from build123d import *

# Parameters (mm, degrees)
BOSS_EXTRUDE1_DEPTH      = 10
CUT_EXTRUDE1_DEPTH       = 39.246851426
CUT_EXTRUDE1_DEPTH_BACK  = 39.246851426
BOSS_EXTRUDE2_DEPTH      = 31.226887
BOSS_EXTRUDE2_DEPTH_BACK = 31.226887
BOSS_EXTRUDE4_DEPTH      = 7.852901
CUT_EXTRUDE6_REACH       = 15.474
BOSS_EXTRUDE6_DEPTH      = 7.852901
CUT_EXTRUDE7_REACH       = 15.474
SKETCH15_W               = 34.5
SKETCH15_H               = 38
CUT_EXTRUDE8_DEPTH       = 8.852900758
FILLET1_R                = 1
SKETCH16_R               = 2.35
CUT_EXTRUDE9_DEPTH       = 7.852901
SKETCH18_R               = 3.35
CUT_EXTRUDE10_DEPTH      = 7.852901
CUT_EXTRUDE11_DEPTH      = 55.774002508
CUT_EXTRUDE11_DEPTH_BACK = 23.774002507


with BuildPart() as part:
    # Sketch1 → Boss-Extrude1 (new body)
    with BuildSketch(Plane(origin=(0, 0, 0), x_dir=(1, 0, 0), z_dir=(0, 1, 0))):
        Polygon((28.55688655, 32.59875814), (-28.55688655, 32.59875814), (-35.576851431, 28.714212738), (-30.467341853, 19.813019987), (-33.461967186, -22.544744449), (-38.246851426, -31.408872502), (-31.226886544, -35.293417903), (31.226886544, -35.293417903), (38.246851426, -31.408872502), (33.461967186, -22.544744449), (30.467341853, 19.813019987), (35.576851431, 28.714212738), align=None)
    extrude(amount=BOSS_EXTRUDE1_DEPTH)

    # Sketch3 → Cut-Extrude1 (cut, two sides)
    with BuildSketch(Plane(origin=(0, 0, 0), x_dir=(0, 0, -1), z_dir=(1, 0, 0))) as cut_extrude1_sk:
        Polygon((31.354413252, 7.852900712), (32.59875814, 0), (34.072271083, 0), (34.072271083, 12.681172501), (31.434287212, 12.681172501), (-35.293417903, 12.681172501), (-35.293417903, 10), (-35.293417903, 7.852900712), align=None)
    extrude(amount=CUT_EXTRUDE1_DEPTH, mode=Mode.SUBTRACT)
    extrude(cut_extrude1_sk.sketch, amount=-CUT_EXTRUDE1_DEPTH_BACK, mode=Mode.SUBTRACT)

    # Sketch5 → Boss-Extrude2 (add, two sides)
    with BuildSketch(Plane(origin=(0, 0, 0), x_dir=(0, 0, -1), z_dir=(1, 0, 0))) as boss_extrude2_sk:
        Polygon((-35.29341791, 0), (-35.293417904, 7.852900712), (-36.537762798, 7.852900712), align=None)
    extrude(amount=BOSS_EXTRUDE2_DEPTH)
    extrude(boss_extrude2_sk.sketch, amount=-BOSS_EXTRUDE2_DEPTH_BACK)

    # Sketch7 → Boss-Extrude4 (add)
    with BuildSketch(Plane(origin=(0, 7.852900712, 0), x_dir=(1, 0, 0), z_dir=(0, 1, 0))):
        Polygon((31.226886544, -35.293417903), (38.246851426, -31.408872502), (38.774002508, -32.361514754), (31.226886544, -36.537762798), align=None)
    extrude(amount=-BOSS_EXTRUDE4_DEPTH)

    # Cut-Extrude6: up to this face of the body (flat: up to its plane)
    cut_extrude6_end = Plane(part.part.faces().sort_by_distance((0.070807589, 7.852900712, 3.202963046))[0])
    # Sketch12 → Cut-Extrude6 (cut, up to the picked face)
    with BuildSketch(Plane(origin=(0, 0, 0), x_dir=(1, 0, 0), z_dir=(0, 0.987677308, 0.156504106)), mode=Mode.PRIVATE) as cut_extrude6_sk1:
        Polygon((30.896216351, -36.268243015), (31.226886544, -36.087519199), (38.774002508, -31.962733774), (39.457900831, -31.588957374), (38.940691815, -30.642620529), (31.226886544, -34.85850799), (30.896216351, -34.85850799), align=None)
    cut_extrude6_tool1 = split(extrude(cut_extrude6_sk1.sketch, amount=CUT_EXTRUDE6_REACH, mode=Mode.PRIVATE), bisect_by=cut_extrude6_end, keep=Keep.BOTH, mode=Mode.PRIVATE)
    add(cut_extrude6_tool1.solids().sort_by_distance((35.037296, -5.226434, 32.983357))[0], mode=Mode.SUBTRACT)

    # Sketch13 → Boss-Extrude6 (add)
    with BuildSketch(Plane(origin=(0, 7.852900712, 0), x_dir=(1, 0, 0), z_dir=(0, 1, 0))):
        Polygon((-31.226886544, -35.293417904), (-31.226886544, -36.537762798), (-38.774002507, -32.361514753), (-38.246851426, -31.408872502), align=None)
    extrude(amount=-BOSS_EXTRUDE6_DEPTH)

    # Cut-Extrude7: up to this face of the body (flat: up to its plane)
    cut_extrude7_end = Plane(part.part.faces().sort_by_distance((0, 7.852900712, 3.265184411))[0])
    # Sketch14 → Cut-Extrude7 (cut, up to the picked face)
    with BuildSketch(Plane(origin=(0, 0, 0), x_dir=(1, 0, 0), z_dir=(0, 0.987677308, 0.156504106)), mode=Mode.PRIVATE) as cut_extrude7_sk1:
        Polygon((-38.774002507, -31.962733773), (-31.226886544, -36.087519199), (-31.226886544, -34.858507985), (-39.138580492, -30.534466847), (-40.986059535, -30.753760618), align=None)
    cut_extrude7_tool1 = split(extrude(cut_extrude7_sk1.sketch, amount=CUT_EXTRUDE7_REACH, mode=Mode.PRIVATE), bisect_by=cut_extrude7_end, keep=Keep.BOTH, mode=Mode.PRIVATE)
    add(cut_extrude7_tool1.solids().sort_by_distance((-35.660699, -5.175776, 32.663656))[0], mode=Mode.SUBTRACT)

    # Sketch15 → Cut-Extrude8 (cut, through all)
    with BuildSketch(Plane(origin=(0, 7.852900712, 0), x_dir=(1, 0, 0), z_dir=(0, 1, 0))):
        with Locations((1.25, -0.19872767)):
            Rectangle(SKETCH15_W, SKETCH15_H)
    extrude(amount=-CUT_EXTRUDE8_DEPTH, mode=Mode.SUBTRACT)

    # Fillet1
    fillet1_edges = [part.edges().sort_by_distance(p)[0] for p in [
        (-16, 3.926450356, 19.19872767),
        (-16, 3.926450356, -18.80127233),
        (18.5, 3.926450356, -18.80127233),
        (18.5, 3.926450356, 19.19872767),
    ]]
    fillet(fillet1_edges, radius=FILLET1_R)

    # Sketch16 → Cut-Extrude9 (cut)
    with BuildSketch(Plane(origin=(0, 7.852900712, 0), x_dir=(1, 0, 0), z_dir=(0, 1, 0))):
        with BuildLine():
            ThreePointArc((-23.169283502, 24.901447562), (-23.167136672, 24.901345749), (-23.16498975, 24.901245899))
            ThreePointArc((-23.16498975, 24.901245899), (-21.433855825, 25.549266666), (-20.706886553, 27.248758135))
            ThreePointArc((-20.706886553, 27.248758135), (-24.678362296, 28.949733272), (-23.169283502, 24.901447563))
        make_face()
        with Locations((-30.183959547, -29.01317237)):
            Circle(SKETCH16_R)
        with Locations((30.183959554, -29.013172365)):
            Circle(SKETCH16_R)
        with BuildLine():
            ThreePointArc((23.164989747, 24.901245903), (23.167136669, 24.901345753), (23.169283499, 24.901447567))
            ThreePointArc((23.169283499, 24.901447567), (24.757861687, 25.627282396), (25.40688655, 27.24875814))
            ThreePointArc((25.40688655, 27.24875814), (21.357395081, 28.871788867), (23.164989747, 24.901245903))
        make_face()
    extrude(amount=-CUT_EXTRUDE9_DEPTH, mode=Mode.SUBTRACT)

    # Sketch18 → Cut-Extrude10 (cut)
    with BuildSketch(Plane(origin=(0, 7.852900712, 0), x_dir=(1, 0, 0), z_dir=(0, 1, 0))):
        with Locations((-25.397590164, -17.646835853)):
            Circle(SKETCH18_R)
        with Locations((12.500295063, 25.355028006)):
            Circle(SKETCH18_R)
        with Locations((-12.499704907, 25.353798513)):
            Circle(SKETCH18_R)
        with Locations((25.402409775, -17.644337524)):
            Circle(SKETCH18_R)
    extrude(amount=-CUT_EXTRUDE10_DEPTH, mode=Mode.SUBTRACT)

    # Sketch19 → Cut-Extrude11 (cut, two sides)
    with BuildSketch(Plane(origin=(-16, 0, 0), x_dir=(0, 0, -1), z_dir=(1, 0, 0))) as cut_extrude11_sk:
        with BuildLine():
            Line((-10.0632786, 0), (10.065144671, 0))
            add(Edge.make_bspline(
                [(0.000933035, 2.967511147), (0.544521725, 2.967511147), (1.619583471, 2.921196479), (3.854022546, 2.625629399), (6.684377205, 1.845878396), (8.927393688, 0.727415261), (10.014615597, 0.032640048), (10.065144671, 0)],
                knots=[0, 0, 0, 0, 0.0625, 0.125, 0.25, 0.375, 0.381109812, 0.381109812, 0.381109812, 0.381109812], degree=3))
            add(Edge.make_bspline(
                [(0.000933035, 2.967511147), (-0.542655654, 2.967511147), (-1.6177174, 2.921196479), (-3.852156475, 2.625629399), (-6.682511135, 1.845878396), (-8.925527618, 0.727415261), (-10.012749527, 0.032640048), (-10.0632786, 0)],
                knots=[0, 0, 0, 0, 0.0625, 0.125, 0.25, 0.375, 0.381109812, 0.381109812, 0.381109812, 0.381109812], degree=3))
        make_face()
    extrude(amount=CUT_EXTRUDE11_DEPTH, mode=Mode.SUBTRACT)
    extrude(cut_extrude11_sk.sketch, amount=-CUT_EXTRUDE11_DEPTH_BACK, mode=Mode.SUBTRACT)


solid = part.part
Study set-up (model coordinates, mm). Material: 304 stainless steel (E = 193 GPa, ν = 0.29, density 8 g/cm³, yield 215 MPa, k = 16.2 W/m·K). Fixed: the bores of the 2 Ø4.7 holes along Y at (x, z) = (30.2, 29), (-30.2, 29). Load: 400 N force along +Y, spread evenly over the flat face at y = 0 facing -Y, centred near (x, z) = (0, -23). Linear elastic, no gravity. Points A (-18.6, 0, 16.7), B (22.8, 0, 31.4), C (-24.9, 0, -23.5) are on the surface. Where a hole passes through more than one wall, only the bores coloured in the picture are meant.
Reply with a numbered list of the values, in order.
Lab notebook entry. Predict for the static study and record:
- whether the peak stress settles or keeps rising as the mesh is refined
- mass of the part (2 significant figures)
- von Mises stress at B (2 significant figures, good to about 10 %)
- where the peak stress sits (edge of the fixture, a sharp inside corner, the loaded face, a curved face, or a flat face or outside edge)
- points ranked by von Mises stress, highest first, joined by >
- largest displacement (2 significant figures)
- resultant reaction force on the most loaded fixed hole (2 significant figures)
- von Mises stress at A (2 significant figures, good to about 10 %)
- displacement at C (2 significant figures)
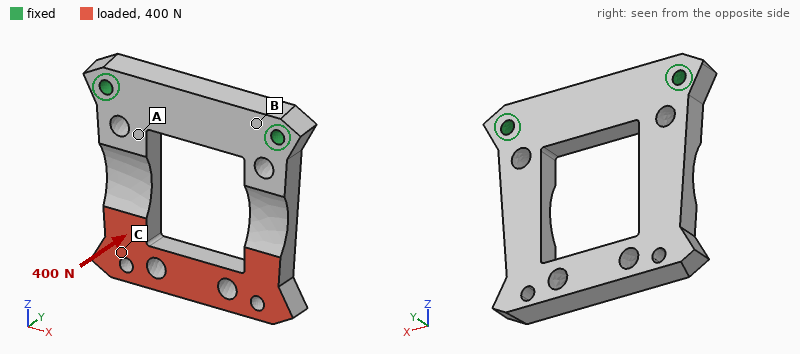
1. keeps rising
2. 180 g
3. 23 MPa
4. edge of the fixture
5. A > B > C
6. 0.18 mm
7. 210 N
8. 64 MPa
9. 0.13 mm
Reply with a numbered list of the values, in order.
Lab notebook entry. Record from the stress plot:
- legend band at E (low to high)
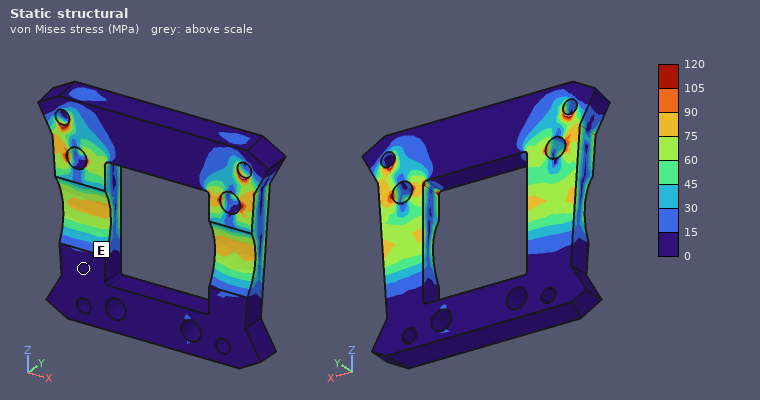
1. 0 to 15 MPa
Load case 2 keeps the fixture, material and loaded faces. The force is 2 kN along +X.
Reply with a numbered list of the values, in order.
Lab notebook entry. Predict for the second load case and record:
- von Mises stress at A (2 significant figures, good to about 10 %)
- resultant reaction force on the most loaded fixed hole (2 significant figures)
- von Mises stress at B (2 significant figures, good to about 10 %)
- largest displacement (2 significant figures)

1. 70 MPa
2. 1.8 kN
3. 22 MPa
4. 75 µm
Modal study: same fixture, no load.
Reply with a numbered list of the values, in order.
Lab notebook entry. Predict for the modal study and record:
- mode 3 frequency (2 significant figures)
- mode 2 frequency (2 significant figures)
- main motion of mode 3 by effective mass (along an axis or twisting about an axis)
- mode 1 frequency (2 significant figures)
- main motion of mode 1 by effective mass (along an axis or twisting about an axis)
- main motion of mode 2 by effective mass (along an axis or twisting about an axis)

1. 4000 Hz
2. 2500 Hz
3. along X
4. 1100 Hz
5. along Y
6. twisting about Z
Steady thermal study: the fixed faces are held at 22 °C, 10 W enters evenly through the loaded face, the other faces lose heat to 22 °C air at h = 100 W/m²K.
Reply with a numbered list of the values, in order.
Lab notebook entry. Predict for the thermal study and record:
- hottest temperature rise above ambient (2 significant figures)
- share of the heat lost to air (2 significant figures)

1. 32 K
2. 94 %
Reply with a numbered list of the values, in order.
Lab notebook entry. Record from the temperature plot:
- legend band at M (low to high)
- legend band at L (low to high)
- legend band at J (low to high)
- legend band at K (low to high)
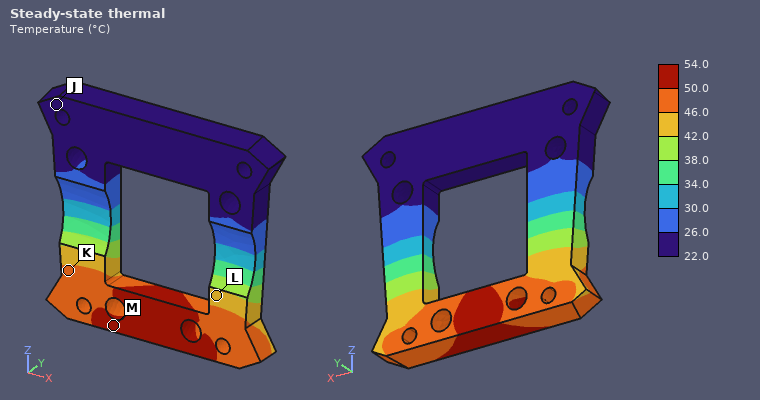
1. 50.0 to 54.0 °C
2. 42.0 to 46.0 °C
3. 22.0 to 26.0 °C
4. 46.0 to 50.0 °C
